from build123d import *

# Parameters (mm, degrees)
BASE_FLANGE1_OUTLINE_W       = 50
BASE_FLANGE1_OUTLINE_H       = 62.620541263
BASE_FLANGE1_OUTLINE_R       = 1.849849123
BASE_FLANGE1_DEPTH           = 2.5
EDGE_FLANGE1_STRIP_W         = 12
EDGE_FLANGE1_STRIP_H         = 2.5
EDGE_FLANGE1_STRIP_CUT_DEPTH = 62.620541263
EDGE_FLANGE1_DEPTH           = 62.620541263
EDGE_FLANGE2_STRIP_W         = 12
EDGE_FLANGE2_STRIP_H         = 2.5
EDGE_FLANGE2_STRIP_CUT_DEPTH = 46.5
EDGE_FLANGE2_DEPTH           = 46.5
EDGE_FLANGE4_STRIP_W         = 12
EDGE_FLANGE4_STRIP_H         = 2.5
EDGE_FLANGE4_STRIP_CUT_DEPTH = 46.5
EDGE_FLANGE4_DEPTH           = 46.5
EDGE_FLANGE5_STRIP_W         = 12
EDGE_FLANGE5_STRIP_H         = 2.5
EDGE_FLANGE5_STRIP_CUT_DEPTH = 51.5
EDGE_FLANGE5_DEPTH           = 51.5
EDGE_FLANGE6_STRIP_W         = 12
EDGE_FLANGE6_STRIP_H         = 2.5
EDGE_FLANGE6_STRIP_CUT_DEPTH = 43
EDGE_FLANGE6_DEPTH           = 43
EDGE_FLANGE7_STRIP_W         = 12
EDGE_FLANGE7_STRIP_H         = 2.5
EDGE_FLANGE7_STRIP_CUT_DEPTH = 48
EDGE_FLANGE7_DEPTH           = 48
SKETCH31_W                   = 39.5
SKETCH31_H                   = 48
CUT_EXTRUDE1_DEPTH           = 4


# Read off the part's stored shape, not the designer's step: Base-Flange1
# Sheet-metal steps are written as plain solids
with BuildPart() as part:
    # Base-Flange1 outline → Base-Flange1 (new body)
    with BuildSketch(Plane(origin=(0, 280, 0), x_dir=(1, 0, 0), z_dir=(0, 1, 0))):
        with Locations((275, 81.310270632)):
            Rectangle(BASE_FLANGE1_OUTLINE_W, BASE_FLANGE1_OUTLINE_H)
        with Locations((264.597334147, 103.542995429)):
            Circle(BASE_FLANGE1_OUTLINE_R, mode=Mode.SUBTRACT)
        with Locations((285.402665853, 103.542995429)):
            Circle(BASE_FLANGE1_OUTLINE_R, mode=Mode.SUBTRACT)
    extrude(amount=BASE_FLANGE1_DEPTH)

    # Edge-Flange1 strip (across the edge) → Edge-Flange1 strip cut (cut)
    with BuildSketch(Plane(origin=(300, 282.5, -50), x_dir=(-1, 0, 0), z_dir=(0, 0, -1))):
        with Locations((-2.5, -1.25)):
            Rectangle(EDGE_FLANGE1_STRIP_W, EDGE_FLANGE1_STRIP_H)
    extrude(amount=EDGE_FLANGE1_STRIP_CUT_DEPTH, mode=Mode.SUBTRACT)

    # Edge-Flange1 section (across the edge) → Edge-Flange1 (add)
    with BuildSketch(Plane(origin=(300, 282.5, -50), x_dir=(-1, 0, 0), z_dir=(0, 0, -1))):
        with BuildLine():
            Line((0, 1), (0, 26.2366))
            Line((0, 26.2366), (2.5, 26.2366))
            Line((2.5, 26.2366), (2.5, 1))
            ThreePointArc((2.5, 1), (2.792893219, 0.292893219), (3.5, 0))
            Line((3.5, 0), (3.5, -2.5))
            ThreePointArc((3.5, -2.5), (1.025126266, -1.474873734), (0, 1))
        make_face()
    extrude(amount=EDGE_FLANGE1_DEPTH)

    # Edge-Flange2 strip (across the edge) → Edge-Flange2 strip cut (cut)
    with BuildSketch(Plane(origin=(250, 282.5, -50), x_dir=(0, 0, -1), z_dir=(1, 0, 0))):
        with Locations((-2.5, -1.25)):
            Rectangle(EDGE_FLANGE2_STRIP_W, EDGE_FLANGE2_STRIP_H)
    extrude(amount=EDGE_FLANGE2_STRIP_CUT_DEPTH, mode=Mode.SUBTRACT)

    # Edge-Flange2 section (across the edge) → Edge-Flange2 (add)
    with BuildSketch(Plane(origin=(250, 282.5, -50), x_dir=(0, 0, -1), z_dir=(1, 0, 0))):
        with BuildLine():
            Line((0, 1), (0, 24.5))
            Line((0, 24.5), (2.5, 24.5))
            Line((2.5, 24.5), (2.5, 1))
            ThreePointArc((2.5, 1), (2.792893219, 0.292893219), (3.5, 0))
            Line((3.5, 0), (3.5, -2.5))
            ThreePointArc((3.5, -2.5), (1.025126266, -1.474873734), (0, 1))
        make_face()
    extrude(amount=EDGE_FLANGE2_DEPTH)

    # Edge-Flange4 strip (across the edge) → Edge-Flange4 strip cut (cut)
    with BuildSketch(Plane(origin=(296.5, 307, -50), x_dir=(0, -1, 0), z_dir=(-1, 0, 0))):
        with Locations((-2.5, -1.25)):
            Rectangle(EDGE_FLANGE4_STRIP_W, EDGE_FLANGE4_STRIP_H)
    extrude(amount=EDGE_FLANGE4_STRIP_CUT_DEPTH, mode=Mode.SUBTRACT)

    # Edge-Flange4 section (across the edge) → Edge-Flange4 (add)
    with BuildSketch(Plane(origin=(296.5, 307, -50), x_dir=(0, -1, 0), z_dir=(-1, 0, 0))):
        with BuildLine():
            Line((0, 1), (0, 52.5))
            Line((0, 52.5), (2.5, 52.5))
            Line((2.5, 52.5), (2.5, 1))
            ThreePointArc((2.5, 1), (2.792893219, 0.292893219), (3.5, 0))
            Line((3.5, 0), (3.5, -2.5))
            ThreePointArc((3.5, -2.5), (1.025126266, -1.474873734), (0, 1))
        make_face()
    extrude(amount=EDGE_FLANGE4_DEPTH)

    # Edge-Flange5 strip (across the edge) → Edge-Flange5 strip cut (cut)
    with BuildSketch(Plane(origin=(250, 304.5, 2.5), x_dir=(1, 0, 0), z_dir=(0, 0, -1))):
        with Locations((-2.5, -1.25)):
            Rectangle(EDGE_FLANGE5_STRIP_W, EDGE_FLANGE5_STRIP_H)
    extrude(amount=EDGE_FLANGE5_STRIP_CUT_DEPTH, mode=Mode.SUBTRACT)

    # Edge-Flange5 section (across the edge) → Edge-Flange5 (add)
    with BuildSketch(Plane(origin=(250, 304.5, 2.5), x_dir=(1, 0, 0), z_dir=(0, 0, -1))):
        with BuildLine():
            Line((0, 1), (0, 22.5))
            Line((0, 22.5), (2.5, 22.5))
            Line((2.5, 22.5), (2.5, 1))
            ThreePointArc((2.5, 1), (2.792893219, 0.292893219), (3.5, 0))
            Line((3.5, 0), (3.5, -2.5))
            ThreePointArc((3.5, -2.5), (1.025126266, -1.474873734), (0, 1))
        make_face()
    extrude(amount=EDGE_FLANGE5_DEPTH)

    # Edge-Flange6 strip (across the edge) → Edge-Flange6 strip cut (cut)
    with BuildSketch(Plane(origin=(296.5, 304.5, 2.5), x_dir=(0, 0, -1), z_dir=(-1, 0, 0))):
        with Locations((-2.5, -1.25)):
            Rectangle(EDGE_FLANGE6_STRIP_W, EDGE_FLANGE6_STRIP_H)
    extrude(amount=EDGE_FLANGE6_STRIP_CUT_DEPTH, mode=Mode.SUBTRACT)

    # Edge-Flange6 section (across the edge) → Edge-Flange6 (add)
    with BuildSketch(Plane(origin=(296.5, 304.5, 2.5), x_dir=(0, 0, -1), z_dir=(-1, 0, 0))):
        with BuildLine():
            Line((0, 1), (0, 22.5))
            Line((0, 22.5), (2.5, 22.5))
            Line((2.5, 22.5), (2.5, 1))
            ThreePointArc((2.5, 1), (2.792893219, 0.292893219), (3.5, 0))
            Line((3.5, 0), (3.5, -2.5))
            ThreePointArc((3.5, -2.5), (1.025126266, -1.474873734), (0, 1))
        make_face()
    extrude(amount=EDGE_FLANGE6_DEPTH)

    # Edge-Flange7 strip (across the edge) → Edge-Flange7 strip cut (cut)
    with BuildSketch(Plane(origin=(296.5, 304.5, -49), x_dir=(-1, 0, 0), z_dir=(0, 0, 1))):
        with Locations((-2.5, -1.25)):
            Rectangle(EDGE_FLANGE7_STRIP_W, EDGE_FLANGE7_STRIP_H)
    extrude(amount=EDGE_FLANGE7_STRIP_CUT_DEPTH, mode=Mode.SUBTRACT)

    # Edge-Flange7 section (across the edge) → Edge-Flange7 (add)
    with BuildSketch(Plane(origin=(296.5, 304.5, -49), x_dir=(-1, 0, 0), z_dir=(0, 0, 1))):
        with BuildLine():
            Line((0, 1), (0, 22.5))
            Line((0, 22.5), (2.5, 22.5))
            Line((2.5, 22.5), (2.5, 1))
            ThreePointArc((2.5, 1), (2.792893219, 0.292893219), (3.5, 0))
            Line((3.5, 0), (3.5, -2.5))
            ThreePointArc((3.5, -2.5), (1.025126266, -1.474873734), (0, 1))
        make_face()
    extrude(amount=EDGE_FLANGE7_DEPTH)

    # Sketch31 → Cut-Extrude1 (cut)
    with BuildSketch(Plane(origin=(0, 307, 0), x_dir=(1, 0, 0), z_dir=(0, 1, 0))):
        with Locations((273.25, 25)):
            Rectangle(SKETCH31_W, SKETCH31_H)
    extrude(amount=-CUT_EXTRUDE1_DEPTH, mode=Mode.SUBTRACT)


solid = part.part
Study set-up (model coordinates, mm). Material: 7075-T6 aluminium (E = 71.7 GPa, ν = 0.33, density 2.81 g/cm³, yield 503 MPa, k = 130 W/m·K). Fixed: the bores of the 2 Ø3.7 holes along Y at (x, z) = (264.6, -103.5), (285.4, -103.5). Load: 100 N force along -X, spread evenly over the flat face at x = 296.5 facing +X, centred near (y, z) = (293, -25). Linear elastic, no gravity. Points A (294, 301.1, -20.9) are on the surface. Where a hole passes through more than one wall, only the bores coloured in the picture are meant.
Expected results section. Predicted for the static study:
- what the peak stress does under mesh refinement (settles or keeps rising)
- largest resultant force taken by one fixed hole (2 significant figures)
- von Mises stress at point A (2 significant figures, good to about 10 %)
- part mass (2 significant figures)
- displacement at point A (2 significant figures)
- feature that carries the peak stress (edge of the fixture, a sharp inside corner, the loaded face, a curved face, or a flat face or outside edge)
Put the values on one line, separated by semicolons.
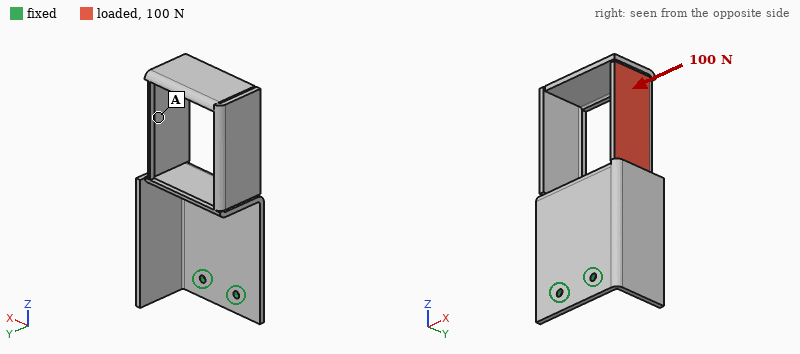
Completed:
keeps rising; 340 N; 18 MPa; 66 g; 0.74 mm; a sharp inside corner
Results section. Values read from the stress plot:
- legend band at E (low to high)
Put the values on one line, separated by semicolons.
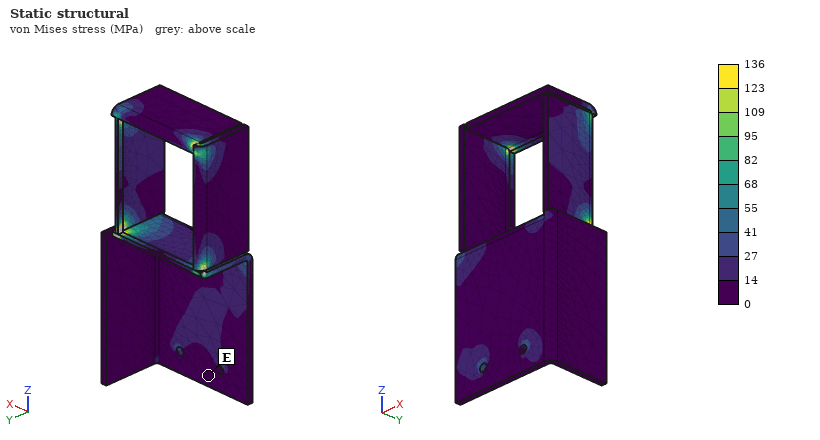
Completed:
0 to 14 MPa
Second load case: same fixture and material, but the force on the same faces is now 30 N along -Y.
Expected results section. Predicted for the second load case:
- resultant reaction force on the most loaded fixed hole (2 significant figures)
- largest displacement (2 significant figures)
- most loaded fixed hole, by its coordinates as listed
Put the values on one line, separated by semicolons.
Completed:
38 N; 1.4 mm; (285.4, -103.5)
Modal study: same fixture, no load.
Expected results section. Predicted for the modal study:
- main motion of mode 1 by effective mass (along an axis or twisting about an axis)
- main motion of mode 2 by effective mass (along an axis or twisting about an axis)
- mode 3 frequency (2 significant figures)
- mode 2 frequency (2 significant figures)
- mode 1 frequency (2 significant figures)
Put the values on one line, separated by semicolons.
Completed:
along Y; along X; 440 Hz; 290 Hz; 150 Hz
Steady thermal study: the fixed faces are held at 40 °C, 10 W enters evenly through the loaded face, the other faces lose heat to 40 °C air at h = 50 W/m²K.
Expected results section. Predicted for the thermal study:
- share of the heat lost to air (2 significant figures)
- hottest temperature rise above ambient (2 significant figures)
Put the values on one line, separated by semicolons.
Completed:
86 %; 45 K
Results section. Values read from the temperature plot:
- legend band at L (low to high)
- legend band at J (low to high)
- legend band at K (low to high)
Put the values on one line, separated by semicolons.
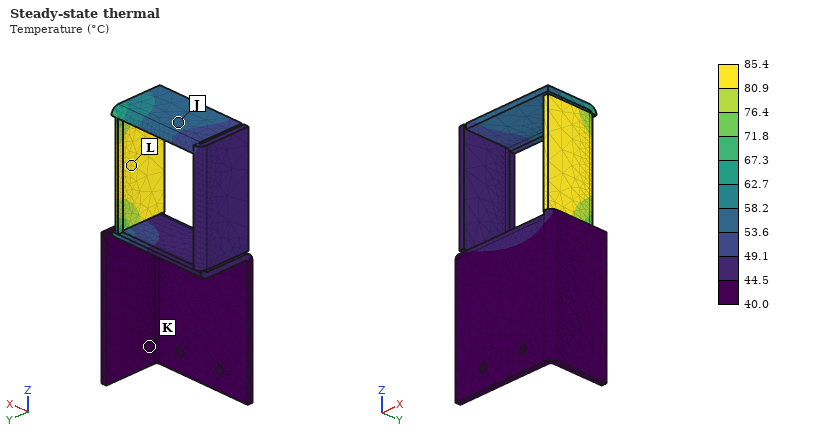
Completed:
80.9 to 85.4 °C; 53.6 to 58.2 °C; 40.0 to 44.5 °C
